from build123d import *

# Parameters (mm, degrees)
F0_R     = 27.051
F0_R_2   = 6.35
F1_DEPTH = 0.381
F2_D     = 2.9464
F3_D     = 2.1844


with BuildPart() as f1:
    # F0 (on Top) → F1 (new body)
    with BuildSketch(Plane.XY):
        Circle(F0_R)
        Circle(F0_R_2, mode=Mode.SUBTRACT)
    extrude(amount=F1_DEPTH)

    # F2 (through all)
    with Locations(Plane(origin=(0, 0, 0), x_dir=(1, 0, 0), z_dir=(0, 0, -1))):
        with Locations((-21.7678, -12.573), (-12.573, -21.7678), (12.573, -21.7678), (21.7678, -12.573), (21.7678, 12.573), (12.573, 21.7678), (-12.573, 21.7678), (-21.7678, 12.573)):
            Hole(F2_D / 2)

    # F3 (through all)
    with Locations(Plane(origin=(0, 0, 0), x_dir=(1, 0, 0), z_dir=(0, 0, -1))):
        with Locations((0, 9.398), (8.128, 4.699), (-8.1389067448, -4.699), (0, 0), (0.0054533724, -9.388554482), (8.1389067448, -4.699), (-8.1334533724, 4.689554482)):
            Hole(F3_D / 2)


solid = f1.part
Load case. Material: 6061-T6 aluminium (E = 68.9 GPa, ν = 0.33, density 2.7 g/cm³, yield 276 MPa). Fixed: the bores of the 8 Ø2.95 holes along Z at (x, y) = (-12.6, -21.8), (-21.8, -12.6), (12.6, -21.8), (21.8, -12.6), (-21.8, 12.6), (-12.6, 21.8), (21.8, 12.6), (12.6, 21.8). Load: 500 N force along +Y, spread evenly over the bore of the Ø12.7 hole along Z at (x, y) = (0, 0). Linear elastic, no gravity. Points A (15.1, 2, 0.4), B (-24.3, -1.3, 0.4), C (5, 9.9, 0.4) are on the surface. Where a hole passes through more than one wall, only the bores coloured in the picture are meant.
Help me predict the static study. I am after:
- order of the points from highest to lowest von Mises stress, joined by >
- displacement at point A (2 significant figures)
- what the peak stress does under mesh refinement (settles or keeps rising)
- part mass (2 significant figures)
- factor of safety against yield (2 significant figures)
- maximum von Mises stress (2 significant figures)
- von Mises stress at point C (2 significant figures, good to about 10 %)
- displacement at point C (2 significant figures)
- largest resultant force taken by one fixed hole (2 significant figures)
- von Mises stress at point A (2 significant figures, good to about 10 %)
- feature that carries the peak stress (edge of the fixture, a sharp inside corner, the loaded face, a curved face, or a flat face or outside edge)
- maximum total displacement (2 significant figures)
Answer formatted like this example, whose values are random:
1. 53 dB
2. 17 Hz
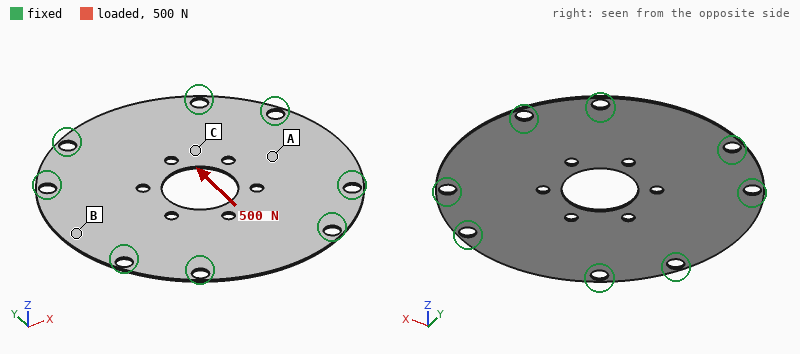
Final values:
1. C > A > B
2. 2.4 µm
3. settles
4. 2.2 g
5. 3.0
6. 94 MPa
7. 28 MPa
8. 6.3 µm
9. 92 N
10. 12 MPa
11. a curved face
12. 9.9 µm
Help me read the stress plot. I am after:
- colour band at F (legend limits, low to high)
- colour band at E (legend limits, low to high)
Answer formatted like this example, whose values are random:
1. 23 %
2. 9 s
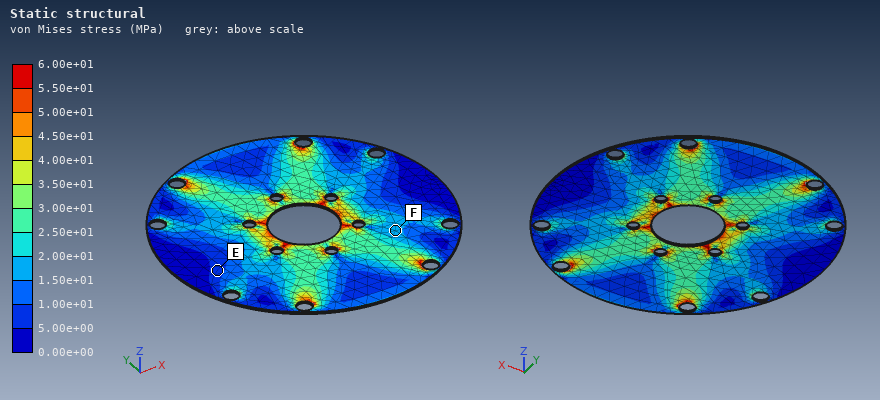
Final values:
1. 1.50e+01 to 2.00e+01 MPa
2. 5.00e+00 to 1.00e+01 MPa
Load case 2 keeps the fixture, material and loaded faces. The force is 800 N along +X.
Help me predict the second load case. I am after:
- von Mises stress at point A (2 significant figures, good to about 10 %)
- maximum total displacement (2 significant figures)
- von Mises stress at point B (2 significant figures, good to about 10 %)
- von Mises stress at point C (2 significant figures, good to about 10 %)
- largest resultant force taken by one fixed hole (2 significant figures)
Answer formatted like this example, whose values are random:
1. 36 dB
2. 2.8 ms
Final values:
1. 27 MPa
2. 15 µm
3. 16 MPa
4. 36 MPa
5. 150 N
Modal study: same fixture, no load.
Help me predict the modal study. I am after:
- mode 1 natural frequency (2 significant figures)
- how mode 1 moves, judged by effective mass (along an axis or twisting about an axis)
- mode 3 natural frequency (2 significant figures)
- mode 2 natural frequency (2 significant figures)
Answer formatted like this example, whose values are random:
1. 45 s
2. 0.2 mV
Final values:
1. 1500 Hz
2. along Z
3. 2700 Hz
4. 2700 Hz
